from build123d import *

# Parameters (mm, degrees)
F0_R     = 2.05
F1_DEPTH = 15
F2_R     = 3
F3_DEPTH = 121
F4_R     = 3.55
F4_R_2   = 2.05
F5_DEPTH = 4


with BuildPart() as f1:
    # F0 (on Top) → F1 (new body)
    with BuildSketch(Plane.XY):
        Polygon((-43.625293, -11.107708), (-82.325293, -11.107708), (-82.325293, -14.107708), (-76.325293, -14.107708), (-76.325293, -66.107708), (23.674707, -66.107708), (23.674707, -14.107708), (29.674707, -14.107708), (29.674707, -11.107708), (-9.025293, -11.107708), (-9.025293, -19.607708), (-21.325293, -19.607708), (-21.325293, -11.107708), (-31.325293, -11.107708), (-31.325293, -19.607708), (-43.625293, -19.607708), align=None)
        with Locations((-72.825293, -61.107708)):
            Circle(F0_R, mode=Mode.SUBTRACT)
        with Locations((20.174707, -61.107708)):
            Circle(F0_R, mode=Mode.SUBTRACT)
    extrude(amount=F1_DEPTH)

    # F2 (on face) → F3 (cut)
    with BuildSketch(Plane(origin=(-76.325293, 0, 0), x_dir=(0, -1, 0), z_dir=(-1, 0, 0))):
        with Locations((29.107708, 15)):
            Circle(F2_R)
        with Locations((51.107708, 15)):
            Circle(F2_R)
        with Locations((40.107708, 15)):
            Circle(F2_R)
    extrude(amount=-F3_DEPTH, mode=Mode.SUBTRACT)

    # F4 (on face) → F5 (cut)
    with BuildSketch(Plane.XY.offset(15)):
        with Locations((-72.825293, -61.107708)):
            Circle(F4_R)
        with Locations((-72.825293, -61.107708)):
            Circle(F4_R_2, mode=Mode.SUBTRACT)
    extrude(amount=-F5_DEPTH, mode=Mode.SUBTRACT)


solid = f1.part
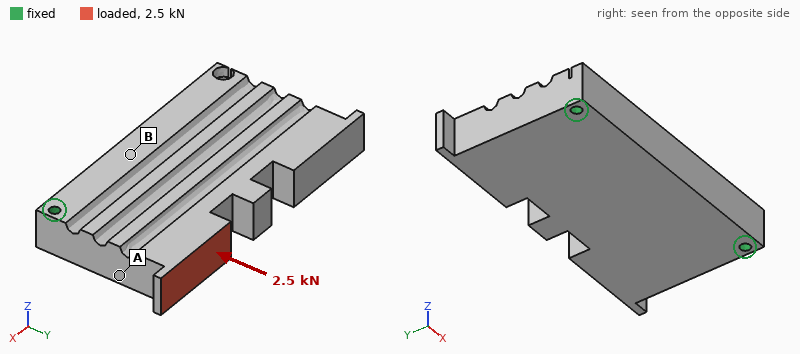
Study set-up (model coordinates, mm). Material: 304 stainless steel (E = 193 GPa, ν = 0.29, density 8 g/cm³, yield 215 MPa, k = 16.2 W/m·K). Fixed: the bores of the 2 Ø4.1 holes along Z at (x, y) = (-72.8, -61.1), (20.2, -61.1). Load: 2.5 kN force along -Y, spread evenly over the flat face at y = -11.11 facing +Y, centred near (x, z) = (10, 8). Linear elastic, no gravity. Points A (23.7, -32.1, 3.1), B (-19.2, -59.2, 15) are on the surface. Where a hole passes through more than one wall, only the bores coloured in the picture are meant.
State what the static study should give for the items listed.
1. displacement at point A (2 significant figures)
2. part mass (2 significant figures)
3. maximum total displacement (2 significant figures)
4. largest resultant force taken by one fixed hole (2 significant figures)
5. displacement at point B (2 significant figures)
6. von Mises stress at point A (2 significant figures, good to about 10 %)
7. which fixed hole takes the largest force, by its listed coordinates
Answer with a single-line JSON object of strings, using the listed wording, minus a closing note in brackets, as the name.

{"displacement at point A": "1.8 µm", "part mass": "600 g", "maximum total displacement": "8.6 µm", "largest resultant force taken by one fixed hole": "2.3 kN", "displacement at point B": "1.4 µm", "von Mises stress at point A": "9.1 MPa", "which fixed hole takes the largest force, by its listed coordinates": "(20.2, -61.1)"}
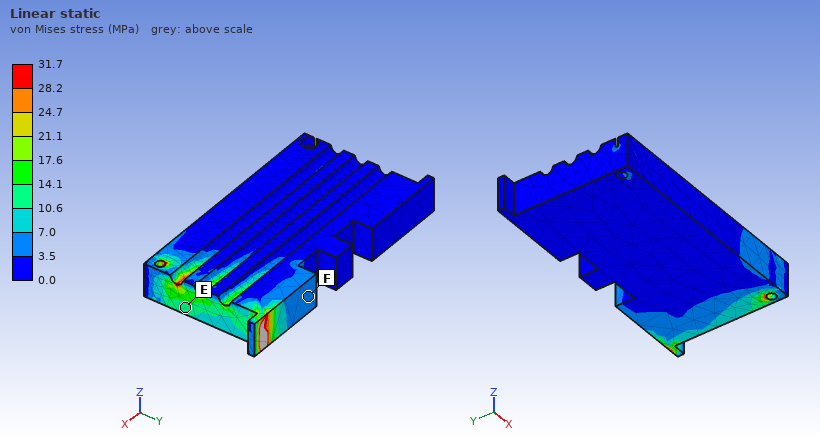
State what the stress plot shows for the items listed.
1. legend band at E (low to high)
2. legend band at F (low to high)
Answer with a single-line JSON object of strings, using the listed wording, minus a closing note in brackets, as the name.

{"legend band at E": "10.6 to 14.1 MPa", "legend band at F": "3.5 to 7.0 MPa"}
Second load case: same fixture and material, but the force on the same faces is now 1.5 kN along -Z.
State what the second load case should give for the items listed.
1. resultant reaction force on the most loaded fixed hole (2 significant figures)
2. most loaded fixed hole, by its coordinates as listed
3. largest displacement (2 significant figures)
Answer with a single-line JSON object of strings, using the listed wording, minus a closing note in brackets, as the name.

{"resultant reaction force on the most loaded fixed hole": "1.4 kN", "most loaded fixed hole, by its coordinates as listed": "(20.2, -61.1)", "largest displacement": "67 µm"}
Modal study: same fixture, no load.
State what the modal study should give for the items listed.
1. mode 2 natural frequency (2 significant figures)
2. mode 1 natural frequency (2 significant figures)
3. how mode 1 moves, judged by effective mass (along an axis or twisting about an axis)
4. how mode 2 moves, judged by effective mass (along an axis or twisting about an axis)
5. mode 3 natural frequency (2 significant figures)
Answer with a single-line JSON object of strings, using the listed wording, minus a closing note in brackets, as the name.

{"mode 2 natural frequency": "4600 Hz", "mode 1 natural frequency": "2100 Hz", "how mode 1 moves, judged by effective mass": "along Z", "how mode 2 moves, judged by effective mass": "twisting about Y", "mode 3 natural frequency": "6200 Hz"}
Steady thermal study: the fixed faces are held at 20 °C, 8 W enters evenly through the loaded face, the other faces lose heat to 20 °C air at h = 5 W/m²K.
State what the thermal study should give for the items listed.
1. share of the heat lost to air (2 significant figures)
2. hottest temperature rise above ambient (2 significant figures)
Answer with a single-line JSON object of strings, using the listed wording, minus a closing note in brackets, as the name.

{"share of the heat lost to air": "16 %", "hottest temperature rise above ambient": "59 K"}
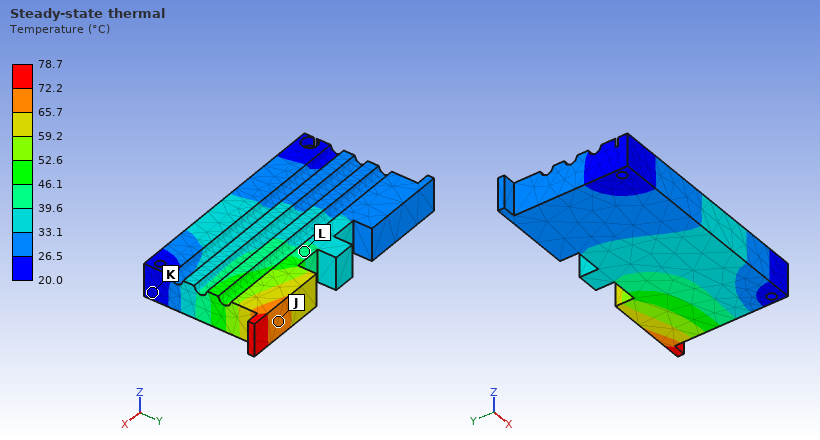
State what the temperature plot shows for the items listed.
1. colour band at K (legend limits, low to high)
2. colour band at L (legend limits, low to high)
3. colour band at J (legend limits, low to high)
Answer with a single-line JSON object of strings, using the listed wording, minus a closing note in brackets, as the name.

{"colour band at K": "20.0 to 26.5 °C", "colour band at L": "39.6 to 46.1 °C", "colour band at J": "65.7 to 72.2 °C"}
